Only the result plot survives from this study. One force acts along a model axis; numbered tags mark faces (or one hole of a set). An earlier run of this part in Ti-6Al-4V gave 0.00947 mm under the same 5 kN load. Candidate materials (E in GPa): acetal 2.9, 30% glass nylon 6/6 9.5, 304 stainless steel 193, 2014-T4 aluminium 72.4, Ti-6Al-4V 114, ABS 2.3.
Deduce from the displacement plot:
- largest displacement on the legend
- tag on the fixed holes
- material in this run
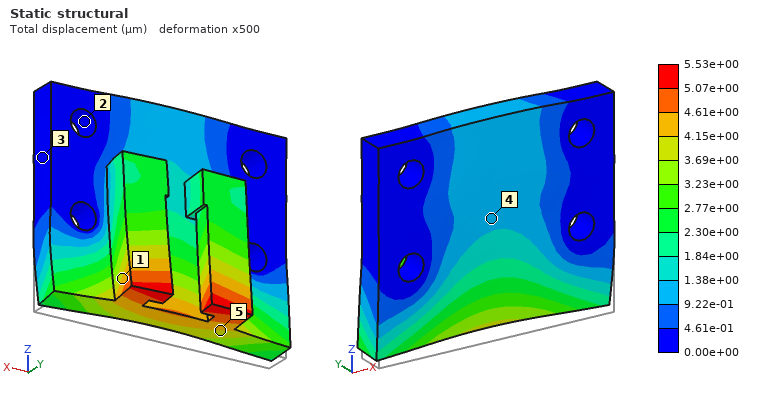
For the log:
5.53e+00 µm
2
304 stainless steel
